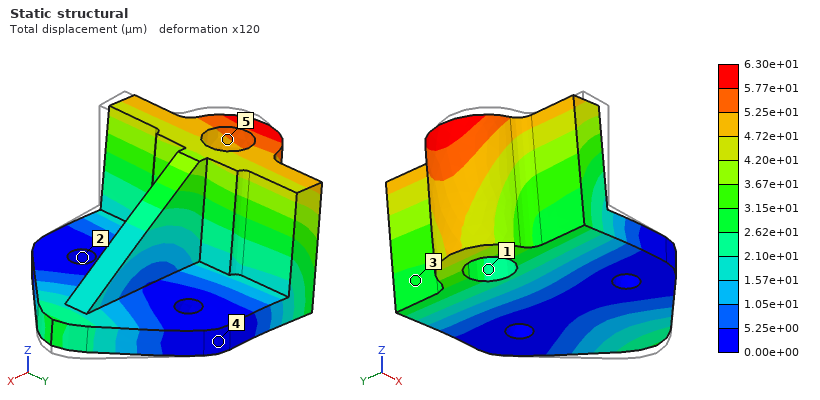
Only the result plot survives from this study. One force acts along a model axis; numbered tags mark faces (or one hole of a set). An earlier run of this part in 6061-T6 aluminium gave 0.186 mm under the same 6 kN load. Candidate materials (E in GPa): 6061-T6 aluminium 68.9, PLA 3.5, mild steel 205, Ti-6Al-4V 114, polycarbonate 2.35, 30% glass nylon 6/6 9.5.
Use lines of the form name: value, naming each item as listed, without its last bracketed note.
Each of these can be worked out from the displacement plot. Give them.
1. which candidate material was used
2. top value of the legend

which candidate material was used: mild steel
top value of the legend: 6.30e+01 µm
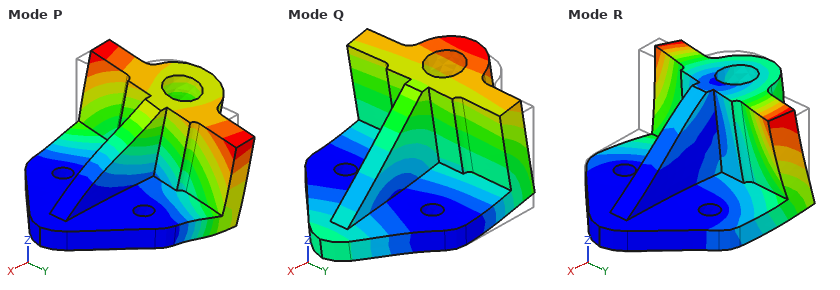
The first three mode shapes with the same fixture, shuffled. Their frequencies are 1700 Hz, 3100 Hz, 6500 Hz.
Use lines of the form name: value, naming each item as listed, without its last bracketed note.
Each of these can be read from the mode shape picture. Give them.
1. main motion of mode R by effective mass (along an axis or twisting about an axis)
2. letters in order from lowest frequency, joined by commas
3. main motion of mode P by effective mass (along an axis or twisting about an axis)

main motion of mode R by effective mass: along Y
letters in order from lowest frequency, joined by commas: Q, P, R
main motion of mode P by effective mass: along Y
